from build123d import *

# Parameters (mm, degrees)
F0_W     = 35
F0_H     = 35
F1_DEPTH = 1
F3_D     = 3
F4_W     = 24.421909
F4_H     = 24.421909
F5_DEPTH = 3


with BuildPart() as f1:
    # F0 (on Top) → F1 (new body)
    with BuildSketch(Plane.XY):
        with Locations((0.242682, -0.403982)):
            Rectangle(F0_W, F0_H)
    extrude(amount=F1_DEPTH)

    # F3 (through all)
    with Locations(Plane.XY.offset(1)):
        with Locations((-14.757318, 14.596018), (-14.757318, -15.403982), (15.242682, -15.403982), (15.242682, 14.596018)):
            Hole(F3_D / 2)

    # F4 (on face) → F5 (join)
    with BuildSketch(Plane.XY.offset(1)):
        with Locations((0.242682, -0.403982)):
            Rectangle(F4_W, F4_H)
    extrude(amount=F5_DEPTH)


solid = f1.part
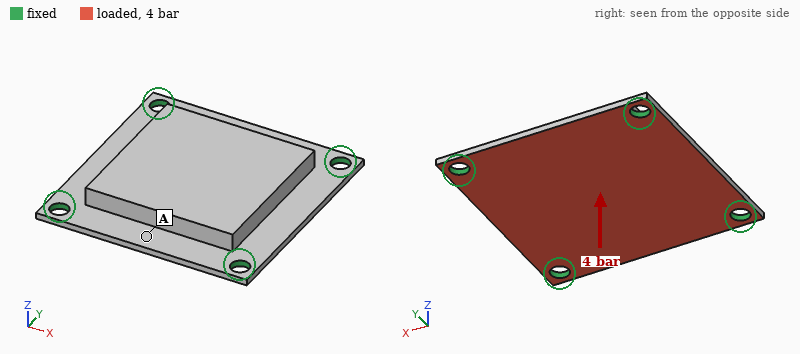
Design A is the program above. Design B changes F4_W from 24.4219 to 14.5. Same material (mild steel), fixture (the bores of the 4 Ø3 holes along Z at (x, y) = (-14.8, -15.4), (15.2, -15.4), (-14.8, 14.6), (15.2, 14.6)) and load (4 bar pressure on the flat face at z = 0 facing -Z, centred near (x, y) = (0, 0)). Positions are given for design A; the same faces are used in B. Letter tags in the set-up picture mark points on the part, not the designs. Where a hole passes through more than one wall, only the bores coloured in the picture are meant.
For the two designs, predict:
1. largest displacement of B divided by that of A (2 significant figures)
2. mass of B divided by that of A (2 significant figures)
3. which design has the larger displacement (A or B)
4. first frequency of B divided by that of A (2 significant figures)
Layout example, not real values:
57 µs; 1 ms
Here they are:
2.8; 0.76; B; 0.63
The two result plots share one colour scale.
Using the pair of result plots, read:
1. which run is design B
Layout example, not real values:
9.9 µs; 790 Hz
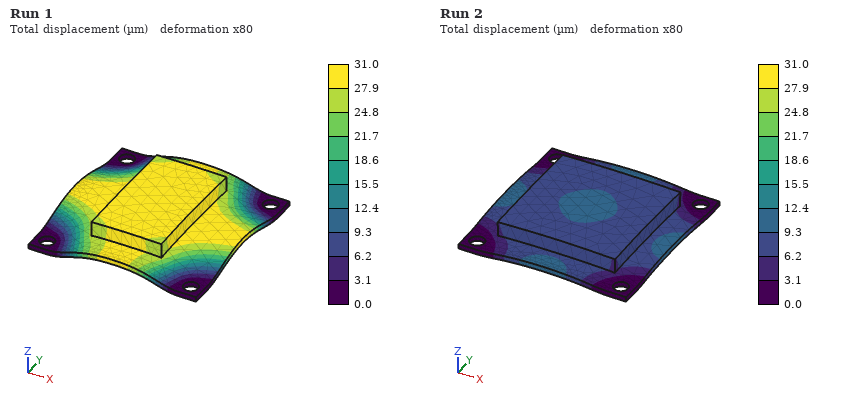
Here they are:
Run 1
